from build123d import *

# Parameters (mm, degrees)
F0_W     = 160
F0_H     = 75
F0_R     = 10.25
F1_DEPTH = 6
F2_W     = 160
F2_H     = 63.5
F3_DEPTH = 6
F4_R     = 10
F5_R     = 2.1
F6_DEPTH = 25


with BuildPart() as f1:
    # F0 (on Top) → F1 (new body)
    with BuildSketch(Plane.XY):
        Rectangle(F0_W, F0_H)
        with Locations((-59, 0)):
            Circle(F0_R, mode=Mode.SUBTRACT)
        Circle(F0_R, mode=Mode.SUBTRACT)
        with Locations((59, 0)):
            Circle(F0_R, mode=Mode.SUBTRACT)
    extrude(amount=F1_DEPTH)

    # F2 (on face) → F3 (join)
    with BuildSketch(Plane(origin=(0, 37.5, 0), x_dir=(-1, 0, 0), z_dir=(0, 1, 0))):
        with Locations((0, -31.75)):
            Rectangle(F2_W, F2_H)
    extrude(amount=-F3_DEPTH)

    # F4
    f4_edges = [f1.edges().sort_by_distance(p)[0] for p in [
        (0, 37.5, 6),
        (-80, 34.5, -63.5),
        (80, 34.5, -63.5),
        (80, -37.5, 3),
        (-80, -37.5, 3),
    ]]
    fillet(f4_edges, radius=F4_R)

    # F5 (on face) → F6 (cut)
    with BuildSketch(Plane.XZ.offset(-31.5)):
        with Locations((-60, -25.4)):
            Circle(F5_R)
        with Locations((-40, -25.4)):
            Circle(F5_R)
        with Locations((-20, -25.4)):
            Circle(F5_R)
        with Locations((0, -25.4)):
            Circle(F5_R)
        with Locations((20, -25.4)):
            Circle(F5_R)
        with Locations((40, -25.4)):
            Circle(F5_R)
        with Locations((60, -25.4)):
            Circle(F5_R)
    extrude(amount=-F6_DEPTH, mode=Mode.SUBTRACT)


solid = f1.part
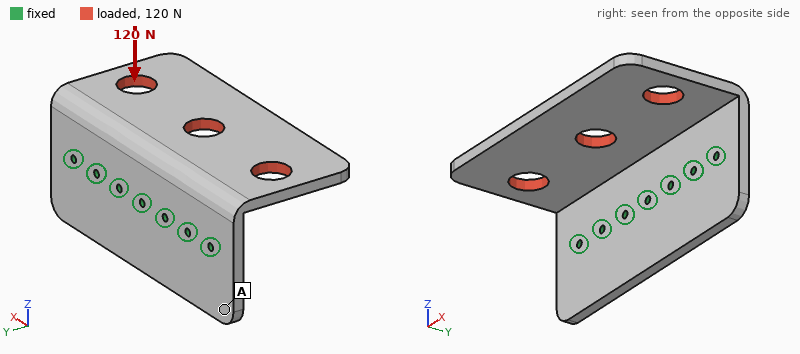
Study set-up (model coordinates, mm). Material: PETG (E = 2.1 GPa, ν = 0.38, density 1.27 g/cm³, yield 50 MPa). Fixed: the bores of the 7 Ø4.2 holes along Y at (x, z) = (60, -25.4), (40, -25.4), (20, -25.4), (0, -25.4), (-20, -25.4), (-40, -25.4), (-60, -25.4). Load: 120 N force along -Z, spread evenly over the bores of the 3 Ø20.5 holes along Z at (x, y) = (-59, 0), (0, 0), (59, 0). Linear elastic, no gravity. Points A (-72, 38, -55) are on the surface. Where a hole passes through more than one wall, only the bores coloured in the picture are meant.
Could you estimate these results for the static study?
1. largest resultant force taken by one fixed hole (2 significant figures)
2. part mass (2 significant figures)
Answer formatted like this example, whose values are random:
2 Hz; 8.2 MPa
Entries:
25 N; 160 g
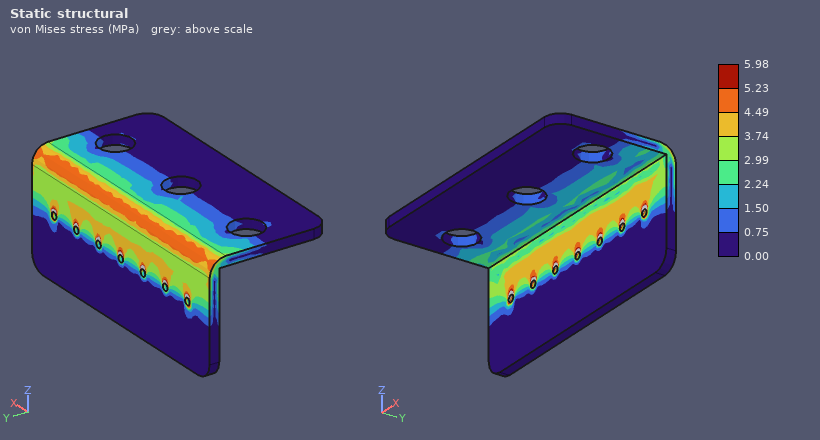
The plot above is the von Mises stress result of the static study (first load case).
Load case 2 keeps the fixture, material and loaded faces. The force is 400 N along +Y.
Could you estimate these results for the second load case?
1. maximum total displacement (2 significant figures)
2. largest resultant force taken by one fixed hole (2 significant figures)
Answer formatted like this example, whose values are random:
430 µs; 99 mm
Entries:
2.0 mm; 63 N
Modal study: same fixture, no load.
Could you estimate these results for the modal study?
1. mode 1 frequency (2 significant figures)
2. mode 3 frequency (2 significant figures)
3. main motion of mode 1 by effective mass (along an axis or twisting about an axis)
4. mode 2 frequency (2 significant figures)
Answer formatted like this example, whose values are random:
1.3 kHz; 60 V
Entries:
150 Hz; 490 Hz; along Z; 250 Hz
